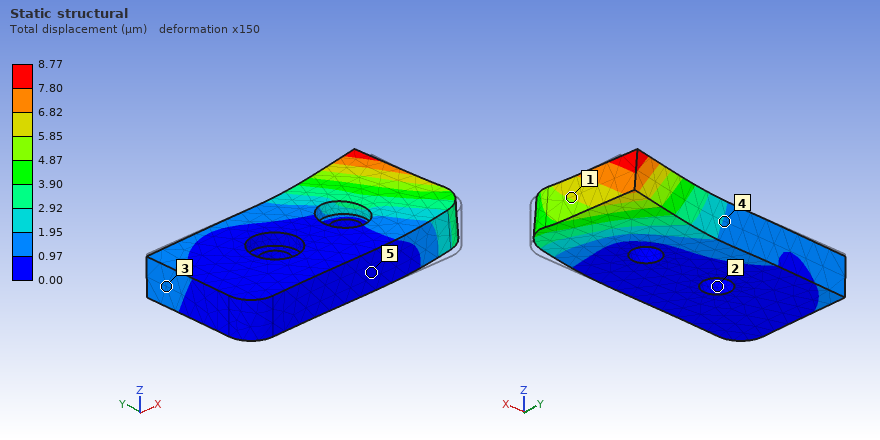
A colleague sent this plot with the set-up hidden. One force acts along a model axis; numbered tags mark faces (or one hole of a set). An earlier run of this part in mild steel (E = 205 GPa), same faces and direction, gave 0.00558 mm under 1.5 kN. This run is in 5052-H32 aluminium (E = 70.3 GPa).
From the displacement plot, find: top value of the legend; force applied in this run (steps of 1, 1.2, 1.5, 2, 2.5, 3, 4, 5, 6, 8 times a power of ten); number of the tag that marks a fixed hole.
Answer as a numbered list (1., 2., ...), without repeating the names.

1. 8.77 µm
2. 800 N
3. 2
